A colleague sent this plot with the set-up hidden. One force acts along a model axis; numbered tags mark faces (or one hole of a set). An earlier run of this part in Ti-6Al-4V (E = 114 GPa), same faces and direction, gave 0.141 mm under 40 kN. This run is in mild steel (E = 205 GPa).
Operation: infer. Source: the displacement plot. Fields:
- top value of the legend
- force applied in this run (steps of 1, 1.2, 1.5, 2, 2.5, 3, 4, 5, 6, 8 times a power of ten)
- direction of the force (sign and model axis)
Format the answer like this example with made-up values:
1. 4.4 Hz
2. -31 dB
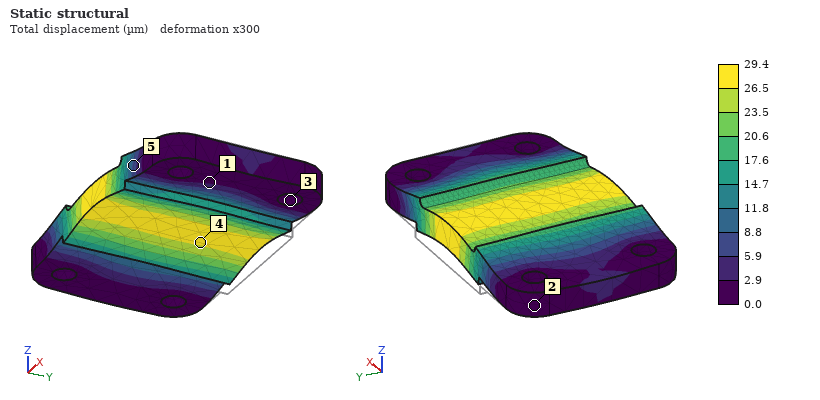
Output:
1. 29.4 µm
2. 15 kN
3. +Z
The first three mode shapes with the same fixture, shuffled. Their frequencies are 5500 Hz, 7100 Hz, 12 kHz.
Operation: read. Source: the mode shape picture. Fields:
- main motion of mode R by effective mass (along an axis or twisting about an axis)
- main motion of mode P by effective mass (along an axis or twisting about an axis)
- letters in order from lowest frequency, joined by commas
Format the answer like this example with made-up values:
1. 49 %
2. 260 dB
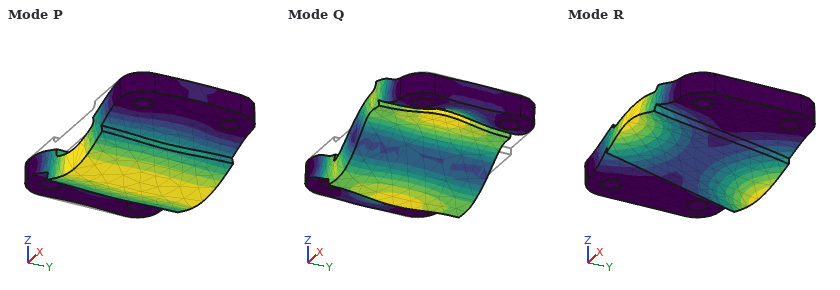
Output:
1. twisting about X
2. along Z
3. P, R, Q
